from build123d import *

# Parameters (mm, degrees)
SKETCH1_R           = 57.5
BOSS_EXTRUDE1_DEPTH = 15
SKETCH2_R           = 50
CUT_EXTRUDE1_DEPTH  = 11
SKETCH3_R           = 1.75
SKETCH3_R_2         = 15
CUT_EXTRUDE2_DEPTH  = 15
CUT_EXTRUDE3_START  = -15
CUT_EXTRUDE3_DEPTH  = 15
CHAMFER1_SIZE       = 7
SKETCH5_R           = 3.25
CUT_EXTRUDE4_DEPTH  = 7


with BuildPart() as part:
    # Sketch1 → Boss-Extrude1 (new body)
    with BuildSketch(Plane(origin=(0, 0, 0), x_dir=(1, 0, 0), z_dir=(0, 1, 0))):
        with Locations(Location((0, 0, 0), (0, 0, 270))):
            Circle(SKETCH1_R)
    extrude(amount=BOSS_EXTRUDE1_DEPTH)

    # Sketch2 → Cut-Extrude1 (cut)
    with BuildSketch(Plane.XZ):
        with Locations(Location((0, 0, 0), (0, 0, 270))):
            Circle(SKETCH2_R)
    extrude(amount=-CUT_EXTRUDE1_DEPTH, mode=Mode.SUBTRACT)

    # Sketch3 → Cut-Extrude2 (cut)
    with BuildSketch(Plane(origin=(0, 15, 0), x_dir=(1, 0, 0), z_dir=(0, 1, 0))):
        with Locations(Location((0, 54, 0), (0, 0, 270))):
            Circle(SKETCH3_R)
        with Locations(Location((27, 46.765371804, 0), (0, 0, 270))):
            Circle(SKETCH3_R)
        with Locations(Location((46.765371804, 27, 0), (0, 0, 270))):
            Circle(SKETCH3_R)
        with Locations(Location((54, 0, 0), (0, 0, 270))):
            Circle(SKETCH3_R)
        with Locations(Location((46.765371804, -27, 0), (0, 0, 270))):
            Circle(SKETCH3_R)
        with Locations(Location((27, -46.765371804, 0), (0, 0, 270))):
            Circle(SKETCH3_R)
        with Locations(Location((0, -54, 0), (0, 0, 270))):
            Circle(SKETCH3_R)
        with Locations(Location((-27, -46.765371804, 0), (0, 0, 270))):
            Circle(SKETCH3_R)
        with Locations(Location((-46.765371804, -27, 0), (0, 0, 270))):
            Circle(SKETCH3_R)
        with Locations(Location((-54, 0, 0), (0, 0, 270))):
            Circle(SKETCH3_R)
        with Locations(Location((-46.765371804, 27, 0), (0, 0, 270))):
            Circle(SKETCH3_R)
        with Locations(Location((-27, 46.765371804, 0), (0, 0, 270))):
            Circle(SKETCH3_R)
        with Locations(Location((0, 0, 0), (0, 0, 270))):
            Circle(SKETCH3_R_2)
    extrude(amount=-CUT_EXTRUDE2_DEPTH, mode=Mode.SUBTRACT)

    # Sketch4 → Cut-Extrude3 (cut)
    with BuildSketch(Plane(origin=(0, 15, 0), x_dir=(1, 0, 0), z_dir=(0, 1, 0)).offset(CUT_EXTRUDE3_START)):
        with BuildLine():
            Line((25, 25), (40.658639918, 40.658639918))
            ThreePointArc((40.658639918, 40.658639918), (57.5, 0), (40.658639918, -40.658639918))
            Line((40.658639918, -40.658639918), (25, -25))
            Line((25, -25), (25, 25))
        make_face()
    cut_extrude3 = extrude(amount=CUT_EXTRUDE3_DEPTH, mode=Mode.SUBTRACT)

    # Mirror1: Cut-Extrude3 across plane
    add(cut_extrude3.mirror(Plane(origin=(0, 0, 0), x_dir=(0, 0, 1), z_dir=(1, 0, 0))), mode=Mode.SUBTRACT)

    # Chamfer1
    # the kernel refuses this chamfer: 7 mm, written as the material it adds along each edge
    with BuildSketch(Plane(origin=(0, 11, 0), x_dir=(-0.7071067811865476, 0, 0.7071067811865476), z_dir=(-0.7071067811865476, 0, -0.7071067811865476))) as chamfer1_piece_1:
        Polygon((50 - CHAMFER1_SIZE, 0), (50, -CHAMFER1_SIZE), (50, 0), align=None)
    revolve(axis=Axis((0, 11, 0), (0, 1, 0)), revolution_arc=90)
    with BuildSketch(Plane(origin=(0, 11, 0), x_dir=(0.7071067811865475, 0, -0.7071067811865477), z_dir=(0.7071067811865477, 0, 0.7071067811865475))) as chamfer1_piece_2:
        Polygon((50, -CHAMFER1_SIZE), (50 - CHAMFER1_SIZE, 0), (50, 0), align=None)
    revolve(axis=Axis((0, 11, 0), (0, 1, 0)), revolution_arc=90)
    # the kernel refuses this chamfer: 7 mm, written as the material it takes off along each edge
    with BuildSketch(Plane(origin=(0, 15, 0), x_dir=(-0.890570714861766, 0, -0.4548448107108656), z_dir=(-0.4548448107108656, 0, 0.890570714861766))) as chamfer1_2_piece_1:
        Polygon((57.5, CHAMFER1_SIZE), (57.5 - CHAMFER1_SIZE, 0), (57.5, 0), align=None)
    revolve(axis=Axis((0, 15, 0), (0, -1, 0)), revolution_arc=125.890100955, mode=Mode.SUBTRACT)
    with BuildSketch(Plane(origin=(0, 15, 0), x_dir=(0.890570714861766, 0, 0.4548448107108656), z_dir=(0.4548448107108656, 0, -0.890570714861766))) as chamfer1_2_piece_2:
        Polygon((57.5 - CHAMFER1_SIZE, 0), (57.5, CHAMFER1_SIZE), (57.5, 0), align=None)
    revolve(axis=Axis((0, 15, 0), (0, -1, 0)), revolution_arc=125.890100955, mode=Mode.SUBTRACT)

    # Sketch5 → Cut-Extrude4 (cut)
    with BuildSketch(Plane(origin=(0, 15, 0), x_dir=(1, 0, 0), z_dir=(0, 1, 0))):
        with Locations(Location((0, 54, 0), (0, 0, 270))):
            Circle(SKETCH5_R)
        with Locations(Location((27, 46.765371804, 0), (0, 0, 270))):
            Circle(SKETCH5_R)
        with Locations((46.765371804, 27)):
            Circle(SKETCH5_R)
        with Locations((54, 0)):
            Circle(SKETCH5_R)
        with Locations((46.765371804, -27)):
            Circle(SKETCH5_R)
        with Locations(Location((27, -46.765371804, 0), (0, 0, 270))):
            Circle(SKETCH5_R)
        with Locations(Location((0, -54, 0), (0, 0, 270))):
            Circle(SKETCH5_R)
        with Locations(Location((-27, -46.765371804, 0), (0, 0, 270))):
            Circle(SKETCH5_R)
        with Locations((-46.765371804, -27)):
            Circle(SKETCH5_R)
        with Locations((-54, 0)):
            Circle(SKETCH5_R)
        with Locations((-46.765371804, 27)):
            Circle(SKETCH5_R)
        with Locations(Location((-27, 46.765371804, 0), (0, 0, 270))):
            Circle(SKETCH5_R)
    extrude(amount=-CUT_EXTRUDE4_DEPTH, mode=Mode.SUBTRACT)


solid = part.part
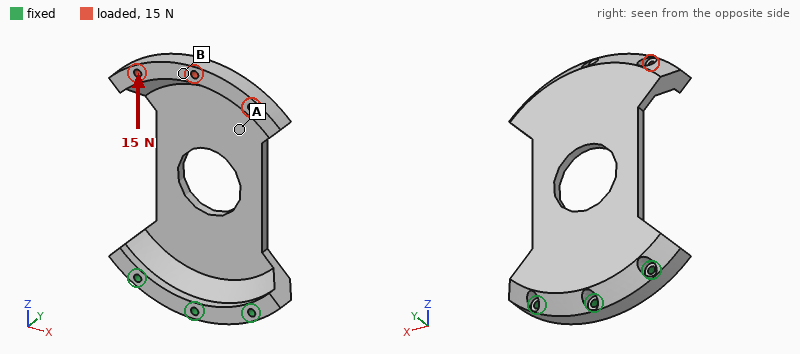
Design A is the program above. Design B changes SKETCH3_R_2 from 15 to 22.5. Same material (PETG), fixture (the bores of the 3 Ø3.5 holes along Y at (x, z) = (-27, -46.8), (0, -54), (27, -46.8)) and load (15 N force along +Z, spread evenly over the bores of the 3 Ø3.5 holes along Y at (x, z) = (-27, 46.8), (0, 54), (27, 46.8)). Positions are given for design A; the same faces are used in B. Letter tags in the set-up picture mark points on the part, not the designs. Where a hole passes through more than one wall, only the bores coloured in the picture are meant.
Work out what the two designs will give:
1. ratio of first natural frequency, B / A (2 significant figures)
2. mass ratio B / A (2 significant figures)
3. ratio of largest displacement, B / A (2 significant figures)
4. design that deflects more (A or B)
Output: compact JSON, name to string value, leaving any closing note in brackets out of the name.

{"ratio of first natural frequency, B / A": "0.67", "mass ratio B / A": "0.90", "ratio of largest displacement, B / A": "2.5", "design that deflects more": "B"}
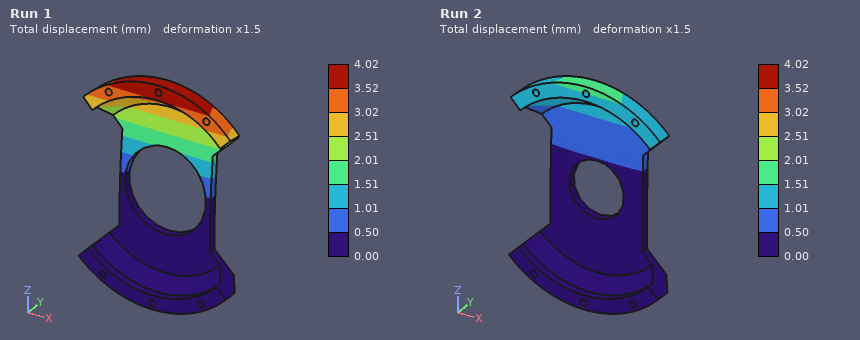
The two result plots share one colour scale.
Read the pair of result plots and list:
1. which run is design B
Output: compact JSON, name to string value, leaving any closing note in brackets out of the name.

{"which run is design B": "Run 1"}
